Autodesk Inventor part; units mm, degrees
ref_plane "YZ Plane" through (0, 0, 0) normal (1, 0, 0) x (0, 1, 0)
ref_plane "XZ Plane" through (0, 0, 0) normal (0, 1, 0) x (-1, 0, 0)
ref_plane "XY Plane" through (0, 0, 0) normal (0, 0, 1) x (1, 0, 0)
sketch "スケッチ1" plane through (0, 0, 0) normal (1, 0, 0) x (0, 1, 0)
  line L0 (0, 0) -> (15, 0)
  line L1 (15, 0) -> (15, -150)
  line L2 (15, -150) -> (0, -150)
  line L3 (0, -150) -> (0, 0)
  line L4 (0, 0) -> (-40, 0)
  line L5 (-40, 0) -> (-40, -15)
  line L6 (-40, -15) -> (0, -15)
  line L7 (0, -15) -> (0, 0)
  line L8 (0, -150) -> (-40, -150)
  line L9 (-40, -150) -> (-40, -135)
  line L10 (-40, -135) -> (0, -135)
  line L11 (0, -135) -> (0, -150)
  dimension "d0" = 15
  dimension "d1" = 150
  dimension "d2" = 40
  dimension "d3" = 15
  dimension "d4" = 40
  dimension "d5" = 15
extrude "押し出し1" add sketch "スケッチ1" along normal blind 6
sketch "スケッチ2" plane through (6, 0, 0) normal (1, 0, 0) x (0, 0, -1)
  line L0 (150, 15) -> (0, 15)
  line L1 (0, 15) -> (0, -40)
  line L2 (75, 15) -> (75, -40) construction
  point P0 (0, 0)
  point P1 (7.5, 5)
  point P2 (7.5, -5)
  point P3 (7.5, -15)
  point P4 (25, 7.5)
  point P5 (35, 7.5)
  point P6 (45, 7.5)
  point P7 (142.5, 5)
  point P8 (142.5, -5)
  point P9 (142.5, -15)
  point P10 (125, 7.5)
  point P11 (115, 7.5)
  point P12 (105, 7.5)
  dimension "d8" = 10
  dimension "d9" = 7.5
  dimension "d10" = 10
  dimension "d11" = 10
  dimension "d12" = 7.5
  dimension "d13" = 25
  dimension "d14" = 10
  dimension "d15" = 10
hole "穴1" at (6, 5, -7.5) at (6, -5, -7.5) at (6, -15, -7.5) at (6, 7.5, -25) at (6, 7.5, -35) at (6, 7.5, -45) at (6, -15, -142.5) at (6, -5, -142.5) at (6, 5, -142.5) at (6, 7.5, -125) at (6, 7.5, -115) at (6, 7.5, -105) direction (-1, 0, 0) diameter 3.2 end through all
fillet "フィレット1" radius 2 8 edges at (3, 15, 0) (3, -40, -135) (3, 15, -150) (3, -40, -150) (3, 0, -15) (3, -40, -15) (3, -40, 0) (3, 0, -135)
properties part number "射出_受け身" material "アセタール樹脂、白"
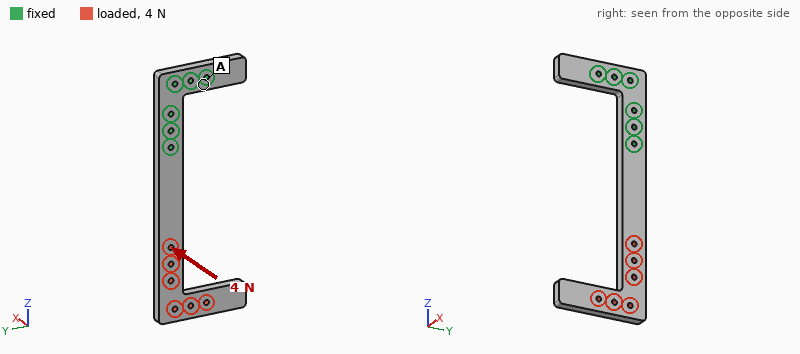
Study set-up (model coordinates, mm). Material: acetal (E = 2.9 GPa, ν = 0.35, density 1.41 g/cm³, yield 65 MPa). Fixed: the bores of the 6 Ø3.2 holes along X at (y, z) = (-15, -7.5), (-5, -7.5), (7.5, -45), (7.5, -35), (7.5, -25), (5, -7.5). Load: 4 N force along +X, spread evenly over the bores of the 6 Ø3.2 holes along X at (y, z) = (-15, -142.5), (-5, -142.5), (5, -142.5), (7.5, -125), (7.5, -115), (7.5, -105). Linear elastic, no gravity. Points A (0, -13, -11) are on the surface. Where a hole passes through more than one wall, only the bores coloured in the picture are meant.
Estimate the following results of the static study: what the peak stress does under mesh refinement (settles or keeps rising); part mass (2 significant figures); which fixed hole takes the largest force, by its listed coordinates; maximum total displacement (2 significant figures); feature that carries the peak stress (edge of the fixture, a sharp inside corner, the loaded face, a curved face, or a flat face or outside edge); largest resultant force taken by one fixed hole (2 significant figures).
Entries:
keeps rising
28 g
(7.5, -45)
1.6 mm
edge of the fixture
14 N
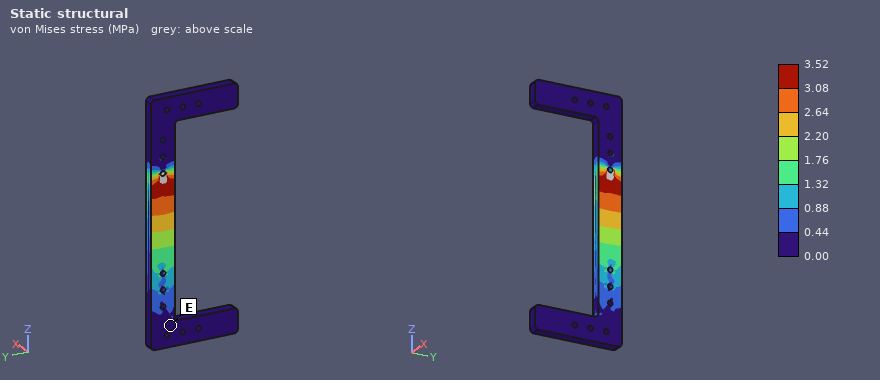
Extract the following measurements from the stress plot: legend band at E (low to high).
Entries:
0.00 to 0.44 MPa
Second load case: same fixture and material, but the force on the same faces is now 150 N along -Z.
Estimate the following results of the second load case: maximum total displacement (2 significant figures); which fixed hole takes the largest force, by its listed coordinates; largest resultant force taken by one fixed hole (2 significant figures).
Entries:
1.5 mm
(7.5, -45)
130 N
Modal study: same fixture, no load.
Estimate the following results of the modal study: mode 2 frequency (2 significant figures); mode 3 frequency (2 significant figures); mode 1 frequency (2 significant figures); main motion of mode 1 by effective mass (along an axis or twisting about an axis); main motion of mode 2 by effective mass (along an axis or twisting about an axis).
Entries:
180 Hz
290 Hz
81 Hz
along X
along Y
